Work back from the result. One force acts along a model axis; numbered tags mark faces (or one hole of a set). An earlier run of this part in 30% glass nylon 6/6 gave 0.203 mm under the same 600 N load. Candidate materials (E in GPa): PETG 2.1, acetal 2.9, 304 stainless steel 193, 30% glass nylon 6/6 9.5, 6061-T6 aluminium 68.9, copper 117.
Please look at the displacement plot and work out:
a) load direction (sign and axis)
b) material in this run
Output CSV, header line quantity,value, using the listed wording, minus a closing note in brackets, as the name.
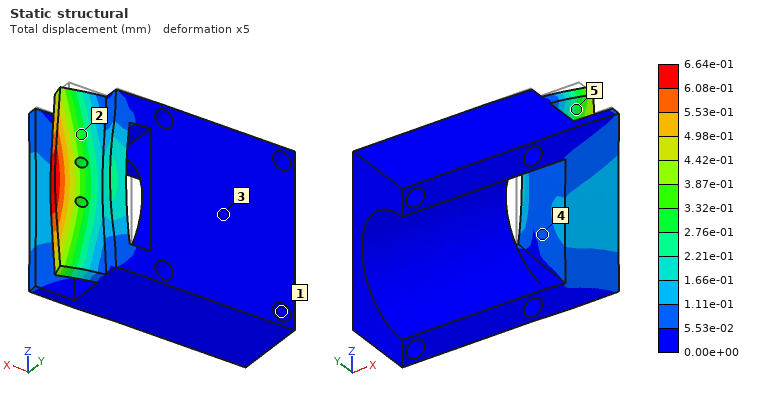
quantity,value
load direction,-Y
material in this run,acetal
